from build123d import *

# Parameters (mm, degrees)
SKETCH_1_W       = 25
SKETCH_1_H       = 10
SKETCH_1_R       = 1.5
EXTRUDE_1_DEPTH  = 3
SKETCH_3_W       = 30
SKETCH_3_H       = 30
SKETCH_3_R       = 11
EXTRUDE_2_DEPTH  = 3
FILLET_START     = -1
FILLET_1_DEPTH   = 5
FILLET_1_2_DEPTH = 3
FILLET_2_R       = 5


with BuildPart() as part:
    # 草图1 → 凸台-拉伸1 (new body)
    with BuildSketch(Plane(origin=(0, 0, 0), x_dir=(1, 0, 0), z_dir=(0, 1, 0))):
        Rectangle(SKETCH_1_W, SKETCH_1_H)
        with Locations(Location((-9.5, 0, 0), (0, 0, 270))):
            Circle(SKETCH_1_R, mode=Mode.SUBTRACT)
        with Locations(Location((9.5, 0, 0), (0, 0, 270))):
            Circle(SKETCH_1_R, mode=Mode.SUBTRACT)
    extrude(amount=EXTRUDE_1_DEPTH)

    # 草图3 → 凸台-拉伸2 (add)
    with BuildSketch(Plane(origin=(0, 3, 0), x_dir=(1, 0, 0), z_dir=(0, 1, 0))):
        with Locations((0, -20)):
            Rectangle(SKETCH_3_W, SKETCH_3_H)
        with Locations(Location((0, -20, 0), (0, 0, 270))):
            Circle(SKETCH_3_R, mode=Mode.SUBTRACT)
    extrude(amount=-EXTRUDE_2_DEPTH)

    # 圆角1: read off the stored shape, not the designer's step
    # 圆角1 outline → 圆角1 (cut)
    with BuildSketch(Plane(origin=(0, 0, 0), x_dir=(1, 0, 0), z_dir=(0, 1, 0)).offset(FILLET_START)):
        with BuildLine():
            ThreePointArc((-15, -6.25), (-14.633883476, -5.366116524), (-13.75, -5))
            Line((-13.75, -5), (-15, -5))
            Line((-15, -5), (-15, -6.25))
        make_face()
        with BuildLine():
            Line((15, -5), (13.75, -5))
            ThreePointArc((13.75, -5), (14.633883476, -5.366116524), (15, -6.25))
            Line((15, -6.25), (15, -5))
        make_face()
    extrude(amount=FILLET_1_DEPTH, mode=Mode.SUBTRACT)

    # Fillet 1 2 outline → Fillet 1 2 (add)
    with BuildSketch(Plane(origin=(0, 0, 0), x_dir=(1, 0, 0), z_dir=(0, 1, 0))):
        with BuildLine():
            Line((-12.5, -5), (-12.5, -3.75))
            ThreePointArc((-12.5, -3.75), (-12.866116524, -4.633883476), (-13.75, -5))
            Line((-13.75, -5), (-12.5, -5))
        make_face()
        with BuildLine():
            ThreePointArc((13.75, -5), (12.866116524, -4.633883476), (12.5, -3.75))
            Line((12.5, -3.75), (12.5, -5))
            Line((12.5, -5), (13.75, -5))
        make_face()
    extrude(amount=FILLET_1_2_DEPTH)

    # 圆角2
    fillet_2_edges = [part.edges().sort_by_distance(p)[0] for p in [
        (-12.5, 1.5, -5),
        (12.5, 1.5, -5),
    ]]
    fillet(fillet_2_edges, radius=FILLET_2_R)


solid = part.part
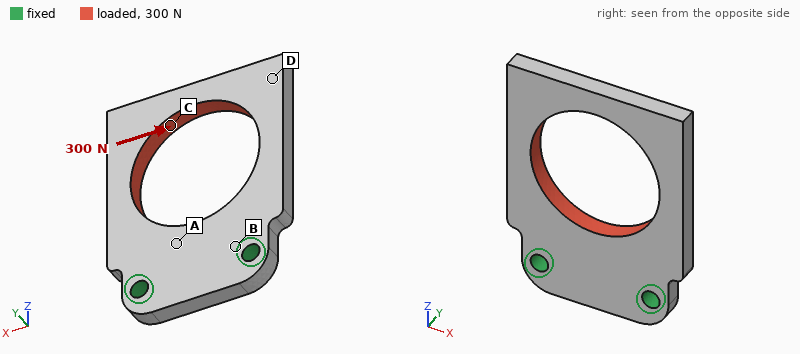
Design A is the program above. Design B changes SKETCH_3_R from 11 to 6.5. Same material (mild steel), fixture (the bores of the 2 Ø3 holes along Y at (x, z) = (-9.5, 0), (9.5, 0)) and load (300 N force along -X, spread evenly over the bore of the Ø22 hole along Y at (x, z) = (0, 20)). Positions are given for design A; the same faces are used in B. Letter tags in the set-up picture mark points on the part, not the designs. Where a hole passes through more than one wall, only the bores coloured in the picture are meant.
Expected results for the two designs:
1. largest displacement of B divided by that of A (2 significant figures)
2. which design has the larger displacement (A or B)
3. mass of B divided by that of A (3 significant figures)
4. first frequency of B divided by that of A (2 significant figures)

0.32
A
1.33
1.1
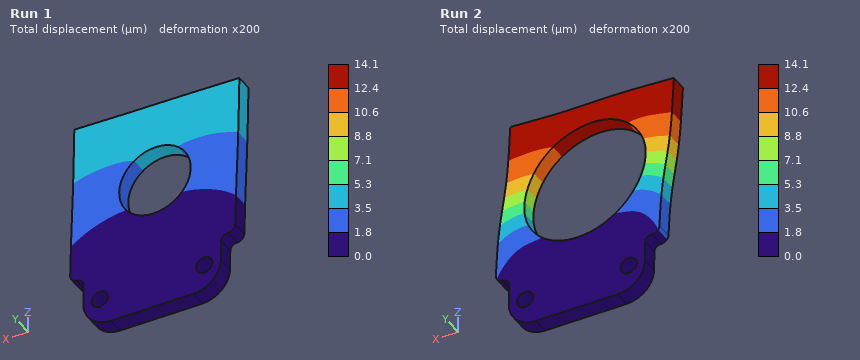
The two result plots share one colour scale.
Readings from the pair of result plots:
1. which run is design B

Run 1
